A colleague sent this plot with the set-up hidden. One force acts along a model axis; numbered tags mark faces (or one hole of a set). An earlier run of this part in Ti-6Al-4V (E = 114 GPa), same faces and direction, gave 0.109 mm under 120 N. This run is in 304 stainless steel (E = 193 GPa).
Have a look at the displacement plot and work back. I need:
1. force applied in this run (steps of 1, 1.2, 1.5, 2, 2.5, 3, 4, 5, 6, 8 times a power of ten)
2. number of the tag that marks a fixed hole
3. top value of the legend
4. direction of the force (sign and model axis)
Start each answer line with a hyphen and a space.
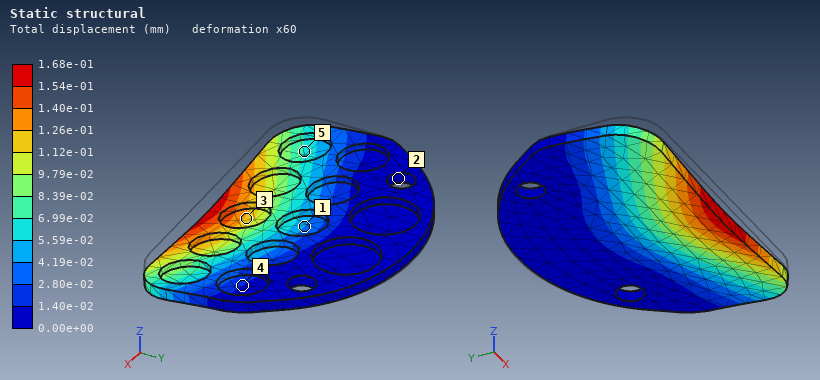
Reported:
- 300 N
- 2
- 1.68e-01 mm
- -Z
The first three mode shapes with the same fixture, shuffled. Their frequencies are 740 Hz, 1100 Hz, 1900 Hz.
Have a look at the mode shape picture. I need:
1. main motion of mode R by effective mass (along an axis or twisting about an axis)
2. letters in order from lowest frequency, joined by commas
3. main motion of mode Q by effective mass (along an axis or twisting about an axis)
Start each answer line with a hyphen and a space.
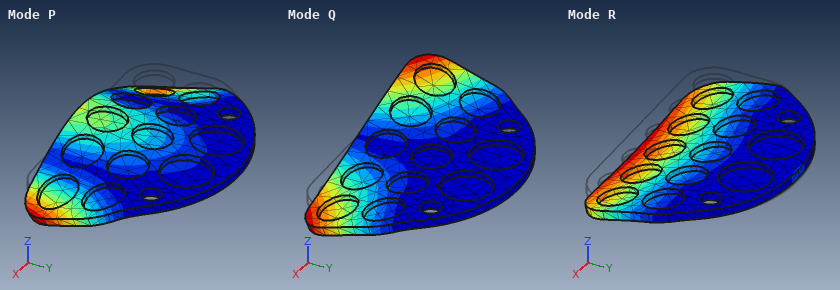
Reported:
- along Z
- R, Q, P
- twisting about Y
